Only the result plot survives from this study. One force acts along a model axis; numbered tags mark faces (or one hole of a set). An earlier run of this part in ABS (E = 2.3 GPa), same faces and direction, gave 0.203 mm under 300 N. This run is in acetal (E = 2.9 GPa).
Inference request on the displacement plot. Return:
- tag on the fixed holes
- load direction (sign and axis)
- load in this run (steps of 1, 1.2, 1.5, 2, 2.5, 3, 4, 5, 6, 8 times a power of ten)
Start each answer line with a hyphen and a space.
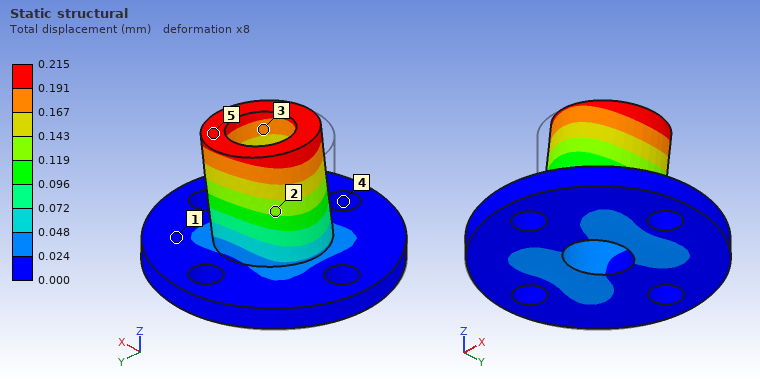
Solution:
- 4
- +X
- 400 N
